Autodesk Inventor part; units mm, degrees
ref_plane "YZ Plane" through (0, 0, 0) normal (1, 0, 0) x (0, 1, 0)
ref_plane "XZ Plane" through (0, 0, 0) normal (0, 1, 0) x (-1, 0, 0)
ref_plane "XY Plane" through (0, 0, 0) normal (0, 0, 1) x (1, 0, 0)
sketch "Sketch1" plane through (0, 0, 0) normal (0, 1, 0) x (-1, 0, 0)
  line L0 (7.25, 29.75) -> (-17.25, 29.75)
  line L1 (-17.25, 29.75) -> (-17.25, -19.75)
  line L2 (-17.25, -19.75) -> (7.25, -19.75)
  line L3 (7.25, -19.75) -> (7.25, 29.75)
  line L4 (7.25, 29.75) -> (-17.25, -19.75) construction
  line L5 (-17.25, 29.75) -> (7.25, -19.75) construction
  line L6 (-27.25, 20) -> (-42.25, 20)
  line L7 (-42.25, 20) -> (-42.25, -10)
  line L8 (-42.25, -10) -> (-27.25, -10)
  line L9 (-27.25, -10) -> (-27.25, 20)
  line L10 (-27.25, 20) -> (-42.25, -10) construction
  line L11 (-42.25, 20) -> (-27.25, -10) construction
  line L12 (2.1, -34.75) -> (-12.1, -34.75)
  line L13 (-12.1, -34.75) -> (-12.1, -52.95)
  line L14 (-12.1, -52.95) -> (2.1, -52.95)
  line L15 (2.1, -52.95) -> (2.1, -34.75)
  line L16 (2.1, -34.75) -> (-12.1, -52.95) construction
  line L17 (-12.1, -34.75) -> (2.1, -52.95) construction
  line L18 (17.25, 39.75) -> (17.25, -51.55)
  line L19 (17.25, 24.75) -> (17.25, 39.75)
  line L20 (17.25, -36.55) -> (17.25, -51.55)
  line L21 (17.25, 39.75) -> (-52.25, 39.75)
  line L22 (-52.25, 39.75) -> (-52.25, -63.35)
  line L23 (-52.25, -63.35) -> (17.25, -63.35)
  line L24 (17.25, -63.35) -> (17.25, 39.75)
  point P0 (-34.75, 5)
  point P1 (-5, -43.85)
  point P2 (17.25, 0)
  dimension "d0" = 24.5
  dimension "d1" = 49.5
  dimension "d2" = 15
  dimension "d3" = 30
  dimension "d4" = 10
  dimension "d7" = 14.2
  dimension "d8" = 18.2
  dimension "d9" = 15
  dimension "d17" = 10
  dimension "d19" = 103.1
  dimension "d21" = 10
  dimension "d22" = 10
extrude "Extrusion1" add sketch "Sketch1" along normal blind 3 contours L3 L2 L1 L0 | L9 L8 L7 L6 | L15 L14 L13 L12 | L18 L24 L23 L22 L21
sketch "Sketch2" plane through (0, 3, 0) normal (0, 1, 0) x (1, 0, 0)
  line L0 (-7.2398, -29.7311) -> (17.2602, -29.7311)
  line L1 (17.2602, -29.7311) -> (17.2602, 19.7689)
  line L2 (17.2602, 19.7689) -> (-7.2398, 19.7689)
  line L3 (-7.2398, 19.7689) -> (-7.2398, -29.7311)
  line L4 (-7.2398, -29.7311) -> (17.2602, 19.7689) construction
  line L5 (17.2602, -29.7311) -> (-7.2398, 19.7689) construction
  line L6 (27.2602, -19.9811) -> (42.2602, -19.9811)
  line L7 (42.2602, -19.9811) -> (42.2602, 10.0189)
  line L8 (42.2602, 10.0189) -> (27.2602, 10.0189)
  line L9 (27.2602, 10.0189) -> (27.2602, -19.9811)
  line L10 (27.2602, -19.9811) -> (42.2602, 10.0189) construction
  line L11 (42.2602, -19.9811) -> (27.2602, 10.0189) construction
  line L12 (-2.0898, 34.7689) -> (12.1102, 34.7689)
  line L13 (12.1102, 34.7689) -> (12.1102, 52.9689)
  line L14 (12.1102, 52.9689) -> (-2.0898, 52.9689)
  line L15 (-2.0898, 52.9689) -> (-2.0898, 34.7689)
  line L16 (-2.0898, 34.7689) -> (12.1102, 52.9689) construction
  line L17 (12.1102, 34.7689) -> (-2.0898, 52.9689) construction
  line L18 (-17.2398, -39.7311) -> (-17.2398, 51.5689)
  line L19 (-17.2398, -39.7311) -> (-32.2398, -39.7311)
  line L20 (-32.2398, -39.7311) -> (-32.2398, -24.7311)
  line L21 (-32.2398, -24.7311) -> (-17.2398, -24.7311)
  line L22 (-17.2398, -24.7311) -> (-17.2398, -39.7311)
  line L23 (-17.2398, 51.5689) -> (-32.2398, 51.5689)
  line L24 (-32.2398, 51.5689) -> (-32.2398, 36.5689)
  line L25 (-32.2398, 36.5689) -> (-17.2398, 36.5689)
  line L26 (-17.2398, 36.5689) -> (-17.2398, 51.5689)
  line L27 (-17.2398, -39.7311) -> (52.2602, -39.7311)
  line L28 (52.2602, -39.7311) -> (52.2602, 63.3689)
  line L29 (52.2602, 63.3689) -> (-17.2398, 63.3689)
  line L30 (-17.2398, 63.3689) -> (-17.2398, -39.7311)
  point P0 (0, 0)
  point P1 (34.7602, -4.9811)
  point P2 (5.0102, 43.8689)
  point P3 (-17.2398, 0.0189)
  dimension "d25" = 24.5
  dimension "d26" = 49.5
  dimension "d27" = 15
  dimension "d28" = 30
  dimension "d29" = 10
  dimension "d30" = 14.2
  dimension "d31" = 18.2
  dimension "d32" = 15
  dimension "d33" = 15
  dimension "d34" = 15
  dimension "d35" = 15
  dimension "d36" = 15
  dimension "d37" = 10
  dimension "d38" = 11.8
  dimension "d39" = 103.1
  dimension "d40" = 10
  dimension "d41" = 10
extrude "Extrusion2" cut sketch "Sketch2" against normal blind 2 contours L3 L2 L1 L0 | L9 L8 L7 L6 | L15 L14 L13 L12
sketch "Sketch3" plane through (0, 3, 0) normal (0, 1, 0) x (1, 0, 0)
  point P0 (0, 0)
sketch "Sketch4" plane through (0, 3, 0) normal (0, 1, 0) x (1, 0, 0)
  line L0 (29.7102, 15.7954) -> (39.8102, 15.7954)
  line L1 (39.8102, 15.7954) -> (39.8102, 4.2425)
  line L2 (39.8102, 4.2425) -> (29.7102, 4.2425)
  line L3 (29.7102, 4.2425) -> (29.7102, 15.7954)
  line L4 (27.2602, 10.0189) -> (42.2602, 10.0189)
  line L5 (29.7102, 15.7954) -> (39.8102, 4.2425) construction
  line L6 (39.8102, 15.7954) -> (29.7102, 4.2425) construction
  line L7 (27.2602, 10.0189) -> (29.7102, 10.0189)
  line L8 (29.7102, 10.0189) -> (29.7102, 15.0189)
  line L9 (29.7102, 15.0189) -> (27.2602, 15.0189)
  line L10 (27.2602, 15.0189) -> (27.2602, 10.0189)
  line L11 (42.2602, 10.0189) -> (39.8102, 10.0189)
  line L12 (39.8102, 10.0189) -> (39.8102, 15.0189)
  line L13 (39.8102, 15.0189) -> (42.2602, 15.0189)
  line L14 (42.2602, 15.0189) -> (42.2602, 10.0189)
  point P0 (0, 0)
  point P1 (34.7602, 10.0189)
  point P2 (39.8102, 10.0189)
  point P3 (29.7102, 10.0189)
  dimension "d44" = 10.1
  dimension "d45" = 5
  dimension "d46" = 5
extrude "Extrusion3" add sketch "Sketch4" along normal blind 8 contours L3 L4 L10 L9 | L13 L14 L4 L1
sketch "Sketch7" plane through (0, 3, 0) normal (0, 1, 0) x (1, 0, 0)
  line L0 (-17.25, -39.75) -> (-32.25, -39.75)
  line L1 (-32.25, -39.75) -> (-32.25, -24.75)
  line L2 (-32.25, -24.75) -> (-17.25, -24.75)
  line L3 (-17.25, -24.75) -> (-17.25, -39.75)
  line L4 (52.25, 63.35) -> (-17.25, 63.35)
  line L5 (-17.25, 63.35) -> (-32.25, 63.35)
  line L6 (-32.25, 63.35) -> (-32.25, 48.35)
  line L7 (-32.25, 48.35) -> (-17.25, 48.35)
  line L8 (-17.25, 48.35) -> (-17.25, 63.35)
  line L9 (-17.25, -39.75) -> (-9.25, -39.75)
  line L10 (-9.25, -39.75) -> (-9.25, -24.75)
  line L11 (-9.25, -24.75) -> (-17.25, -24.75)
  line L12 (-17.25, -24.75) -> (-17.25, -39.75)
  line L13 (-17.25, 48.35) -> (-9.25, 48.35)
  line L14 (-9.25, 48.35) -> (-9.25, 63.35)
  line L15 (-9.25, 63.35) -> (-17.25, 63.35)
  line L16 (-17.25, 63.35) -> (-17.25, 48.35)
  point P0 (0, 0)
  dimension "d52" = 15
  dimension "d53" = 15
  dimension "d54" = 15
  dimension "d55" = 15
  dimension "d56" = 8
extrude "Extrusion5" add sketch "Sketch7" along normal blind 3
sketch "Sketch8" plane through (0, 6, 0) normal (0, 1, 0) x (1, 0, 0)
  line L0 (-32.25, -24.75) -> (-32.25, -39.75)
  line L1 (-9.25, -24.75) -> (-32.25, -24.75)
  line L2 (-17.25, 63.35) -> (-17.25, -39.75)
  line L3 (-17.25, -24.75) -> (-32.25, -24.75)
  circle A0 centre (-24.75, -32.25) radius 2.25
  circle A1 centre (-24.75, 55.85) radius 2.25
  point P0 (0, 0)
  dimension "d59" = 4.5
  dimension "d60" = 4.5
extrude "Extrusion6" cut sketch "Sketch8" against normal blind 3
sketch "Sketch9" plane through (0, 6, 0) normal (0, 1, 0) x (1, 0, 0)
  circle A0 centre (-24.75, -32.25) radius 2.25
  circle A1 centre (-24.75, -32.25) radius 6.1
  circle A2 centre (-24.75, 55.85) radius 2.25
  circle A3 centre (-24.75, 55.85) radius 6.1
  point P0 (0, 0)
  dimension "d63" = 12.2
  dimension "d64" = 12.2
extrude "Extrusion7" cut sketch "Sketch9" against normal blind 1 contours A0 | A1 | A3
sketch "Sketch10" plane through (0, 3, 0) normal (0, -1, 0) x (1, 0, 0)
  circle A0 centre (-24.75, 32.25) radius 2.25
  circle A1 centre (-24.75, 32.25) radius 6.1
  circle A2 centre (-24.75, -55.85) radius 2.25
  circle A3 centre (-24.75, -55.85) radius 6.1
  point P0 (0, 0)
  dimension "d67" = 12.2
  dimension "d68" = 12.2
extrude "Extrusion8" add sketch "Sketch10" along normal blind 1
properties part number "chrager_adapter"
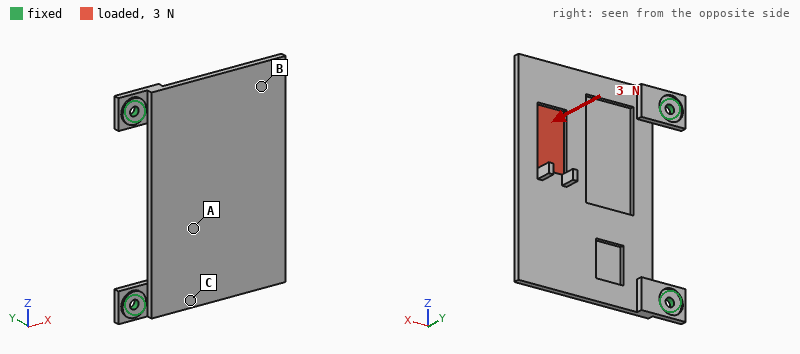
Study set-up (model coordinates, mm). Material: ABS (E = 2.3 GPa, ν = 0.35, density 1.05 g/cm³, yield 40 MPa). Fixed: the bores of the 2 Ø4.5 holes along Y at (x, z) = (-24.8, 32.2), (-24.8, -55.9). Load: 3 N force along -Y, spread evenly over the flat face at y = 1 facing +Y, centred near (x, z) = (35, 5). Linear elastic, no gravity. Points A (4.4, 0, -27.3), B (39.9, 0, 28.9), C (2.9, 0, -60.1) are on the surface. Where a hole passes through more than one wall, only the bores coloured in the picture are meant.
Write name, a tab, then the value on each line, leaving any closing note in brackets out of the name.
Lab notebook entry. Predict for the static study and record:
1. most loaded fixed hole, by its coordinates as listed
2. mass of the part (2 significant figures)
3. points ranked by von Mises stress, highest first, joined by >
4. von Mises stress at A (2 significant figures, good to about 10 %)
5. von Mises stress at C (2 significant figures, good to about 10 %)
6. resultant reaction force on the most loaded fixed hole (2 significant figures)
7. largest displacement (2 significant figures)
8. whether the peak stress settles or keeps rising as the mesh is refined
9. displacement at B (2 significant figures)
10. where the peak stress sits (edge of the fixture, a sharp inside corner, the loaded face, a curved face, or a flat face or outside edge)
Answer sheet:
most loaded fixed hole, by its coordinates as listed	(-24.8, 32.2)
mass of the part	21 g
points ranked by von Mises stress, highest first, joined by >	C > A > B
von Mises stress at A	0.81 MPa
von Mises stress at C	1.4 MPa
resultant reaction force on the most loaded fixed hole	2.1 N
largest displacement	1.5 mm
whether the peak stress settles or keeps rising as the mesh is refined	keeps rising
displacement at B	1.2 mm
where the peak stress sits	edge of the fixture
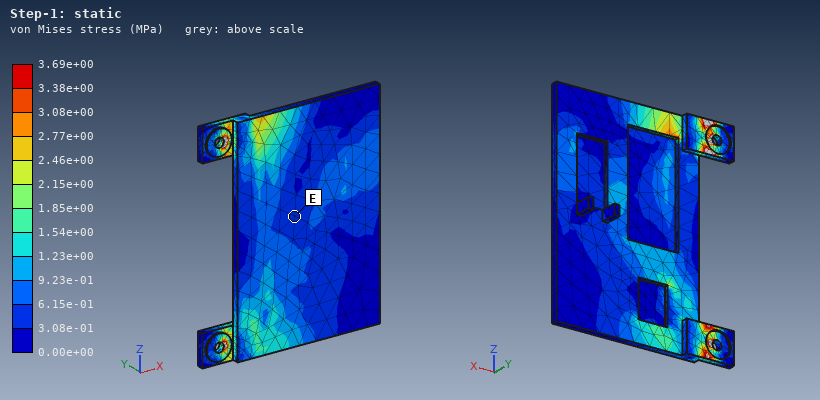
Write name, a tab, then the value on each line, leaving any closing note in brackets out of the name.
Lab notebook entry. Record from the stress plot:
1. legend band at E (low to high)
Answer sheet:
legend band at E	3.08e-01 to 6.15e-01 MPa
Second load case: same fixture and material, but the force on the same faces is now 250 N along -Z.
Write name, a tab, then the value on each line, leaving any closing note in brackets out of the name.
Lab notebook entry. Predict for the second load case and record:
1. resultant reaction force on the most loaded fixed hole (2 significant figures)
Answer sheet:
resultant reaction force on the most loaded fixed hole	200 N
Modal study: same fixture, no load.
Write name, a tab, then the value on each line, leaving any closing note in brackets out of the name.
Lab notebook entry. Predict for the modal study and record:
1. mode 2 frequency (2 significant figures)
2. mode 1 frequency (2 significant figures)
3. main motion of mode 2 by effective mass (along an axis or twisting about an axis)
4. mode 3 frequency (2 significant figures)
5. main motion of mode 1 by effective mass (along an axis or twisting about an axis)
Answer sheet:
mode 2 frequency	210 Hz
mode 1 frequency	81 Hz
main motion of mode 2 by effective mass	twisting about X
mode 3 frequency	480 Hz
main motion of mode 1 by effective mass	along Y
